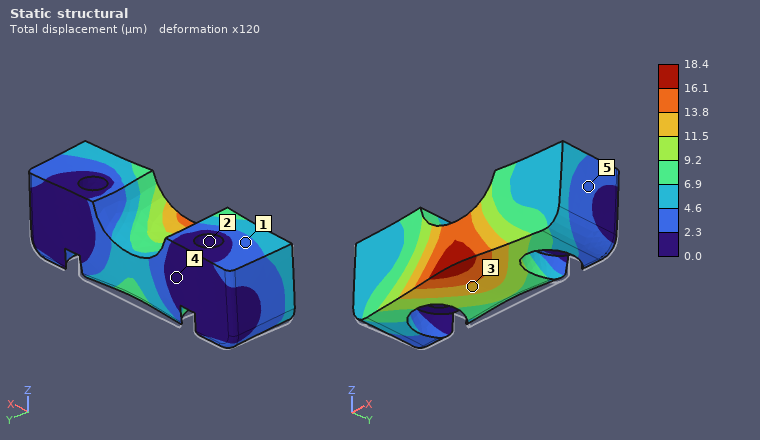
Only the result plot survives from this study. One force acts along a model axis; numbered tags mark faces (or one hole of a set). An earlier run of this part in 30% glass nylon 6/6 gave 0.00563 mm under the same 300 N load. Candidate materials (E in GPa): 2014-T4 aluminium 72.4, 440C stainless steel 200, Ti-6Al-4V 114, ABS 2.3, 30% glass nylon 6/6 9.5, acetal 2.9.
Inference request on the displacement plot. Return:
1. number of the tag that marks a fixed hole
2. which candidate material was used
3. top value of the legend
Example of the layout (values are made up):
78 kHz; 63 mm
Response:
2; acetal; 18.4 µm
